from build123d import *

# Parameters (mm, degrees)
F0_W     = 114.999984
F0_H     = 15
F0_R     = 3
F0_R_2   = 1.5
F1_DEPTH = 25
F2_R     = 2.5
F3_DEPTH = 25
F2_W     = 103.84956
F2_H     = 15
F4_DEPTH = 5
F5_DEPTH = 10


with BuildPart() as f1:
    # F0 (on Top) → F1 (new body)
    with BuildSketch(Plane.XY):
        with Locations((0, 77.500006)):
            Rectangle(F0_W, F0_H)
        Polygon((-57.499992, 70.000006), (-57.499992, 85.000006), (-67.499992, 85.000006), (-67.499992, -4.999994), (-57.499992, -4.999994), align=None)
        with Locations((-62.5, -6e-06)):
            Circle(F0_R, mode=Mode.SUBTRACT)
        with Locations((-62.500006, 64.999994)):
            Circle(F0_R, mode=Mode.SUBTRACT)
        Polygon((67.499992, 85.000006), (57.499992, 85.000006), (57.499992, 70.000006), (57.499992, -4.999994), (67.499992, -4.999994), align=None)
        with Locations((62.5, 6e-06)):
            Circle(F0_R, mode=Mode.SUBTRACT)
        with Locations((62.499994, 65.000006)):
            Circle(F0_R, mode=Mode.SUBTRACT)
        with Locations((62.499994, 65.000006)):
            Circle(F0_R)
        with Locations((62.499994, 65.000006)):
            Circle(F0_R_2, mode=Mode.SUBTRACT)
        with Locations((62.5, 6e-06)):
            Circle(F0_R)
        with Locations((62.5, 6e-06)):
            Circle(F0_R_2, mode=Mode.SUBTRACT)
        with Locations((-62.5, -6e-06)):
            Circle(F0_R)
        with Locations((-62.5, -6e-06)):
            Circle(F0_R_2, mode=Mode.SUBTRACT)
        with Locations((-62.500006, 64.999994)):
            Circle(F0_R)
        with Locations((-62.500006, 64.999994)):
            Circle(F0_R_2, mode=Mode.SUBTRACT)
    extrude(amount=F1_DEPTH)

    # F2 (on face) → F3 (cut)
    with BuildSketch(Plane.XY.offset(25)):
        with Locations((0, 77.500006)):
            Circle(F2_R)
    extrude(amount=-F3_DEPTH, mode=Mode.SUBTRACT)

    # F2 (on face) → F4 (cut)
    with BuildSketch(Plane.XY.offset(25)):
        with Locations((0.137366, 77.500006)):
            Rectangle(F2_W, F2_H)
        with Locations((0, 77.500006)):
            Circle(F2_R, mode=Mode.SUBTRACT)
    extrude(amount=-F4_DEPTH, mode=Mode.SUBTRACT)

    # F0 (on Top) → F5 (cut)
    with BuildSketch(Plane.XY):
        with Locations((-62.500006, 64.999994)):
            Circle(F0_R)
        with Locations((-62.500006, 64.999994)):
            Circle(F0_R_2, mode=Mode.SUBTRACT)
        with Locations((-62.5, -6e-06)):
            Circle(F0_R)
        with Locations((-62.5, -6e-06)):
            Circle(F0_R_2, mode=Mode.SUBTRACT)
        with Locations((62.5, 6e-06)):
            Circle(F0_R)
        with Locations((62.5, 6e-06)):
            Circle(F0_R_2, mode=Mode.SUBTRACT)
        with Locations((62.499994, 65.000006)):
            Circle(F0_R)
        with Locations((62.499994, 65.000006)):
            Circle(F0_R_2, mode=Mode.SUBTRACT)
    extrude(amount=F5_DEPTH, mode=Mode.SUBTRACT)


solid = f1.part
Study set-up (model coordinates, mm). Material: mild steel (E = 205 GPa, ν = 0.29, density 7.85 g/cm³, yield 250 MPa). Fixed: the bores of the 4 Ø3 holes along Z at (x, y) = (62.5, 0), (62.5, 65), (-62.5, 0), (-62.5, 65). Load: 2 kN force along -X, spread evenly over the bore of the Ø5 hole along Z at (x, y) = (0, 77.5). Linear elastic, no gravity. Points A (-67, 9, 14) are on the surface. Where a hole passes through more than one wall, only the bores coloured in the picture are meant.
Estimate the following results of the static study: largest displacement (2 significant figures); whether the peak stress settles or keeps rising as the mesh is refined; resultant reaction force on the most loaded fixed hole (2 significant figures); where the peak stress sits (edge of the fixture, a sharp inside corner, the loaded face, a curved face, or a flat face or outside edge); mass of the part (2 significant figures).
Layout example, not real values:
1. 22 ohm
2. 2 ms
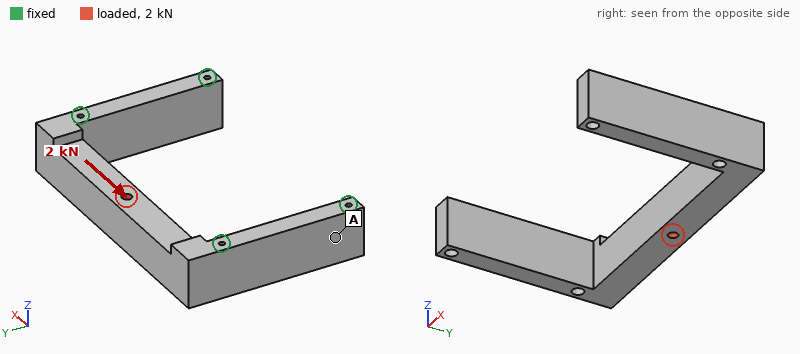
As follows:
1. 3.5 µm
2. keeps rising
3. 1.0 kN
4. edge of the fixture
5. 620 g
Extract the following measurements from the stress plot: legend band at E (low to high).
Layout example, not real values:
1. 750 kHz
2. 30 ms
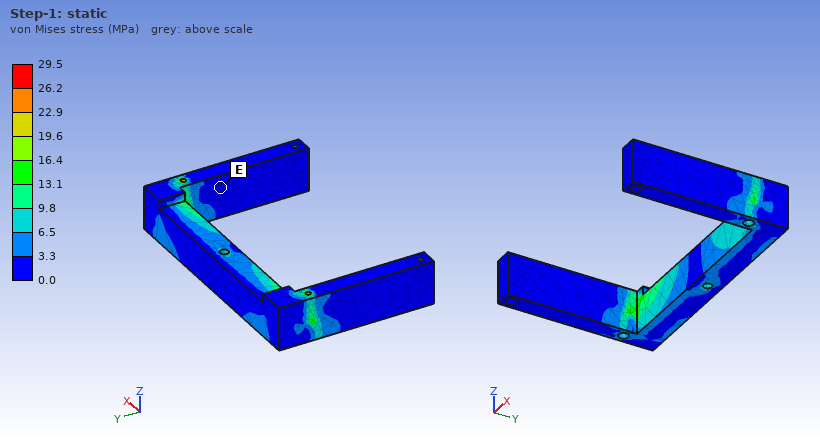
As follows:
1. 0.0 to 3.3 MPa
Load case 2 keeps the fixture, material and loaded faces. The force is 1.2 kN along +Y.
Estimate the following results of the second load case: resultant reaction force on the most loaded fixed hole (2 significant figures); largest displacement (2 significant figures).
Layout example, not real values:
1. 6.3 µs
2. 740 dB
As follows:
1. 1.1 kN
2. 18 µm
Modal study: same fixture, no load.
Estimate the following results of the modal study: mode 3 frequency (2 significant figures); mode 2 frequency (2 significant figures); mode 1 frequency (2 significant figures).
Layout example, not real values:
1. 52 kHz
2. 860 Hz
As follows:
1. 6600 Hz
2. 4300 Hz
3. 3500 Hz
